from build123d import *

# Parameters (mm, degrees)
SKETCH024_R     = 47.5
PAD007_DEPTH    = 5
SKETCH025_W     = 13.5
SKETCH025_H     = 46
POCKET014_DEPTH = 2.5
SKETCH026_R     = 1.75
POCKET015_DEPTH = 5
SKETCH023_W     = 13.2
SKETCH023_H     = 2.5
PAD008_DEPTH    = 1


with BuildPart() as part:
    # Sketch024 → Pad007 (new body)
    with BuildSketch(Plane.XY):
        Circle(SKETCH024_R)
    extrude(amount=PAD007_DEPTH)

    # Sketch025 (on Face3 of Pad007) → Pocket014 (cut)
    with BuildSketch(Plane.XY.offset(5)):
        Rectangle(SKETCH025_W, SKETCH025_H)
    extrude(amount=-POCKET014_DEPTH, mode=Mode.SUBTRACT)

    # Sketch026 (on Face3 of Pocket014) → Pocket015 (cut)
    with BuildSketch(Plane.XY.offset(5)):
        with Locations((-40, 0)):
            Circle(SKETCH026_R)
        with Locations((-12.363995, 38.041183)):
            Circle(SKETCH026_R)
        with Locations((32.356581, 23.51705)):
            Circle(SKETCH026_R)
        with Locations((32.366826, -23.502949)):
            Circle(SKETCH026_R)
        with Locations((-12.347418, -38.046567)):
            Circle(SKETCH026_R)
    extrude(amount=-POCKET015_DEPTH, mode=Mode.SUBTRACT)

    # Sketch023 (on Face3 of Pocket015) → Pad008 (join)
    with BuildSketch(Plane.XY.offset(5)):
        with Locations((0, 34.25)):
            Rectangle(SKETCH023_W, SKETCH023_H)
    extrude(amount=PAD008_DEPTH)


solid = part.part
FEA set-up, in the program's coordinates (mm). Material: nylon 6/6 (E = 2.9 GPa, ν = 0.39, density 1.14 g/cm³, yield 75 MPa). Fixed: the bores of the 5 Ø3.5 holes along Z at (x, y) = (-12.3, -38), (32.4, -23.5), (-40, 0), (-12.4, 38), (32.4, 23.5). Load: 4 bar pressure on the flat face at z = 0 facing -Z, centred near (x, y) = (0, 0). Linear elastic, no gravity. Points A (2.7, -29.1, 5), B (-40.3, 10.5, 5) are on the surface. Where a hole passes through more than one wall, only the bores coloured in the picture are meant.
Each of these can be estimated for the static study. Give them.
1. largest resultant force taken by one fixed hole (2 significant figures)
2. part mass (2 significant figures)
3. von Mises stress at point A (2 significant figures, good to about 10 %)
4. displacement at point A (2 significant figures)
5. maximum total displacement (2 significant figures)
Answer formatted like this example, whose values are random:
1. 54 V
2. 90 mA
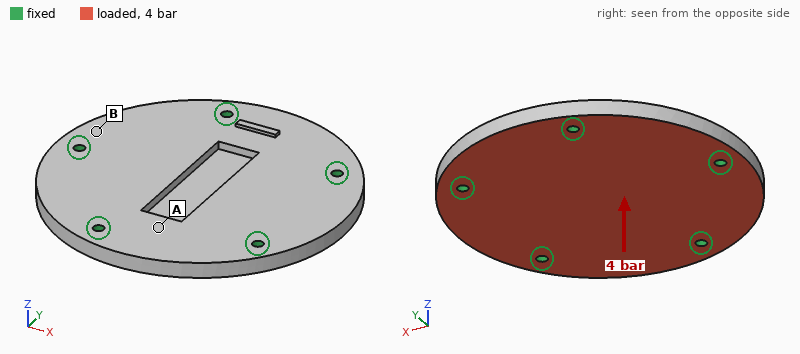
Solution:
1. 590 N
2. 38 g
3. 15 MPa
4. 0.39 mm
5. 1.1 mm
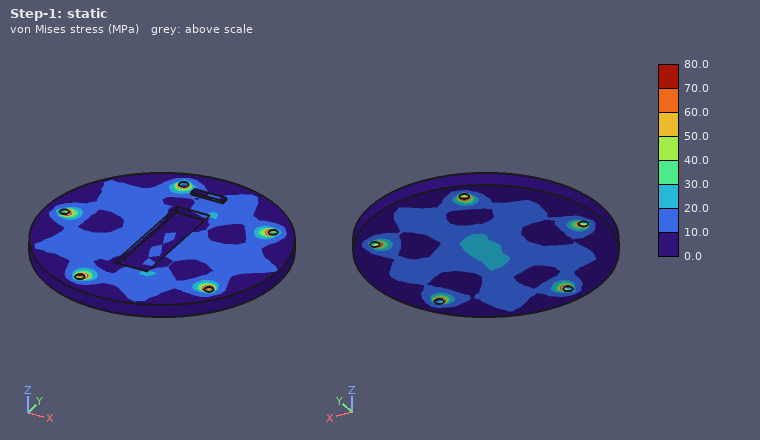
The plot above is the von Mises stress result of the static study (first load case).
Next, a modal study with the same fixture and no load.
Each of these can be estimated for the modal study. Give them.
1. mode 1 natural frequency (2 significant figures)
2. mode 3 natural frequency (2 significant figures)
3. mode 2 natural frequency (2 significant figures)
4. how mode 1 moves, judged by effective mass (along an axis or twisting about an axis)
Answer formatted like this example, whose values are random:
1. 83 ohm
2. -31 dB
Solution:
1. 1800 Hz
2. 2700 Hz
3. 2700 Hz
4. along Z
